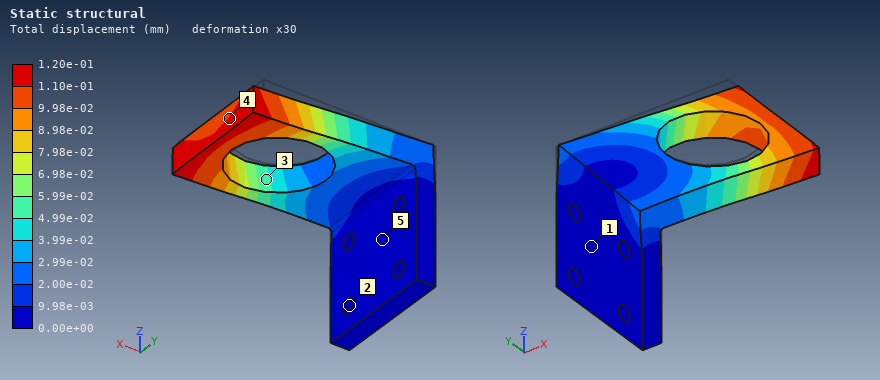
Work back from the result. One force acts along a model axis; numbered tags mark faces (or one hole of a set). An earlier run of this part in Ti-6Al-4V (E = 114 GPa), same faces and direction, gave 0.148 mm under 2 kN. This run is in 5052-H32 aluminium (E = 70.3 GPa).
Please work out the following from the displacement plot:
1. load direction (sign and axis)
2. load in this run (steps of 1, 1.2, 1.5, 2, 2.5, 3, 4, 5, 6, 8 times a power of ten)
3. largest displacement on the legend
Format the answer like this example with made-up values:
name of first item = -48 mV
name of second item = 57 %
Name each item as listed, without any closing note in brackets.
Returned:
load direction = -Y
load in this run = 1 kN
largest displacement on the legend = 1.20e-01 mm
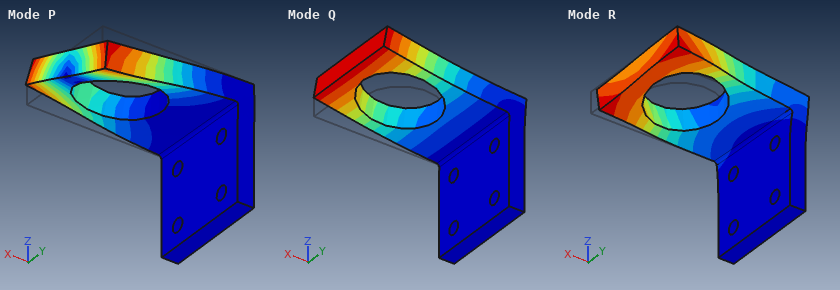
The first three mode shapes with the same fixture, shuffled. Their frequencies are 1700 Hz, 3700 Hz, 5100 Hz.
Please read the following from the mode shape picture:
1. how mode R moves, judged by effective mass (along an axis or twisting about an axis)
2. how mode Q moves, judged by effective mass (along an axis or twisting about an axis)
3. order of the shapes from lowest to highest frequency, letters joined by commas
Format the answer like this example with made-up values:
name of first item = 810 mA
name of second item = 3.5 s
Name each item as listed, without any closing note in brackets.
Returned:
how mode R moves, judged by effective mass = along Y
how mode Q moves, judged by effective mass = along Z
order of the shapes from lowest to highest frequency, letters joined by commas = Q, R, P
